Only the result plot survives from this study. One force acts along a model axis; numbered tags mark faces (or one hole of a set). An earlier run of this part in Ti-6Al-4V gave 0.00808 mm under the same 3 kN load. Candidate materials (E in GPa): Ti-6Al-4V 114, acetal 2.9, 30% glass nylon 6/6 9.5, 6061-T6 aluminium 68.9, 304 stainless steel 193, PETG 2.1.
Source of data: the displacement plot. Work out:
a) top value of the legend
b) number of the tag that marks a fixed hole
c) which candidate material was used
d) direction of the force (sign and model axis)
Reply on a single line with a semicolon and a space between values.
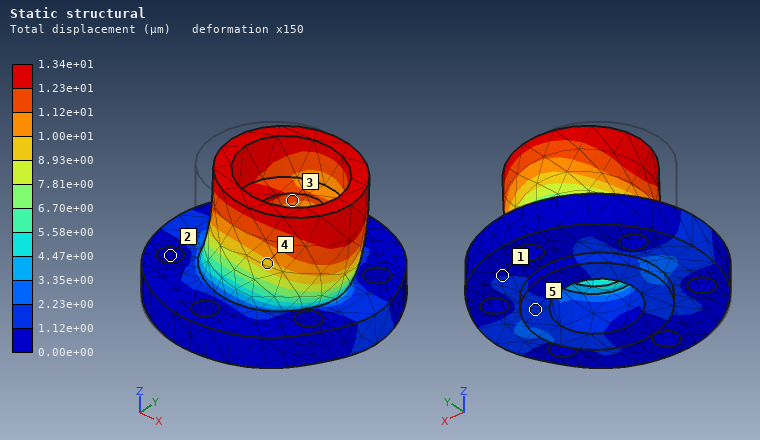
1.34e+01 µm; 2; 6061-T6 aluminium; +X
